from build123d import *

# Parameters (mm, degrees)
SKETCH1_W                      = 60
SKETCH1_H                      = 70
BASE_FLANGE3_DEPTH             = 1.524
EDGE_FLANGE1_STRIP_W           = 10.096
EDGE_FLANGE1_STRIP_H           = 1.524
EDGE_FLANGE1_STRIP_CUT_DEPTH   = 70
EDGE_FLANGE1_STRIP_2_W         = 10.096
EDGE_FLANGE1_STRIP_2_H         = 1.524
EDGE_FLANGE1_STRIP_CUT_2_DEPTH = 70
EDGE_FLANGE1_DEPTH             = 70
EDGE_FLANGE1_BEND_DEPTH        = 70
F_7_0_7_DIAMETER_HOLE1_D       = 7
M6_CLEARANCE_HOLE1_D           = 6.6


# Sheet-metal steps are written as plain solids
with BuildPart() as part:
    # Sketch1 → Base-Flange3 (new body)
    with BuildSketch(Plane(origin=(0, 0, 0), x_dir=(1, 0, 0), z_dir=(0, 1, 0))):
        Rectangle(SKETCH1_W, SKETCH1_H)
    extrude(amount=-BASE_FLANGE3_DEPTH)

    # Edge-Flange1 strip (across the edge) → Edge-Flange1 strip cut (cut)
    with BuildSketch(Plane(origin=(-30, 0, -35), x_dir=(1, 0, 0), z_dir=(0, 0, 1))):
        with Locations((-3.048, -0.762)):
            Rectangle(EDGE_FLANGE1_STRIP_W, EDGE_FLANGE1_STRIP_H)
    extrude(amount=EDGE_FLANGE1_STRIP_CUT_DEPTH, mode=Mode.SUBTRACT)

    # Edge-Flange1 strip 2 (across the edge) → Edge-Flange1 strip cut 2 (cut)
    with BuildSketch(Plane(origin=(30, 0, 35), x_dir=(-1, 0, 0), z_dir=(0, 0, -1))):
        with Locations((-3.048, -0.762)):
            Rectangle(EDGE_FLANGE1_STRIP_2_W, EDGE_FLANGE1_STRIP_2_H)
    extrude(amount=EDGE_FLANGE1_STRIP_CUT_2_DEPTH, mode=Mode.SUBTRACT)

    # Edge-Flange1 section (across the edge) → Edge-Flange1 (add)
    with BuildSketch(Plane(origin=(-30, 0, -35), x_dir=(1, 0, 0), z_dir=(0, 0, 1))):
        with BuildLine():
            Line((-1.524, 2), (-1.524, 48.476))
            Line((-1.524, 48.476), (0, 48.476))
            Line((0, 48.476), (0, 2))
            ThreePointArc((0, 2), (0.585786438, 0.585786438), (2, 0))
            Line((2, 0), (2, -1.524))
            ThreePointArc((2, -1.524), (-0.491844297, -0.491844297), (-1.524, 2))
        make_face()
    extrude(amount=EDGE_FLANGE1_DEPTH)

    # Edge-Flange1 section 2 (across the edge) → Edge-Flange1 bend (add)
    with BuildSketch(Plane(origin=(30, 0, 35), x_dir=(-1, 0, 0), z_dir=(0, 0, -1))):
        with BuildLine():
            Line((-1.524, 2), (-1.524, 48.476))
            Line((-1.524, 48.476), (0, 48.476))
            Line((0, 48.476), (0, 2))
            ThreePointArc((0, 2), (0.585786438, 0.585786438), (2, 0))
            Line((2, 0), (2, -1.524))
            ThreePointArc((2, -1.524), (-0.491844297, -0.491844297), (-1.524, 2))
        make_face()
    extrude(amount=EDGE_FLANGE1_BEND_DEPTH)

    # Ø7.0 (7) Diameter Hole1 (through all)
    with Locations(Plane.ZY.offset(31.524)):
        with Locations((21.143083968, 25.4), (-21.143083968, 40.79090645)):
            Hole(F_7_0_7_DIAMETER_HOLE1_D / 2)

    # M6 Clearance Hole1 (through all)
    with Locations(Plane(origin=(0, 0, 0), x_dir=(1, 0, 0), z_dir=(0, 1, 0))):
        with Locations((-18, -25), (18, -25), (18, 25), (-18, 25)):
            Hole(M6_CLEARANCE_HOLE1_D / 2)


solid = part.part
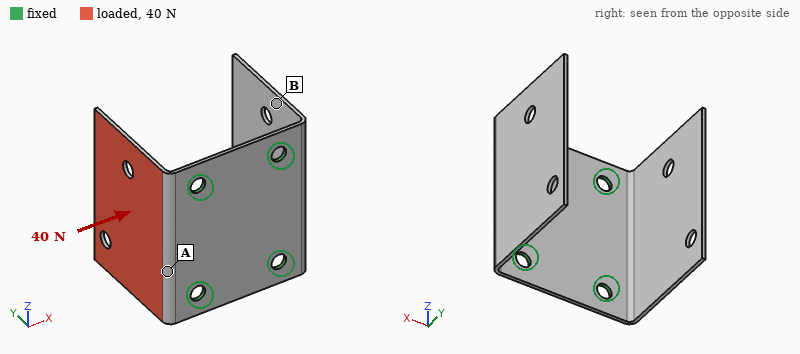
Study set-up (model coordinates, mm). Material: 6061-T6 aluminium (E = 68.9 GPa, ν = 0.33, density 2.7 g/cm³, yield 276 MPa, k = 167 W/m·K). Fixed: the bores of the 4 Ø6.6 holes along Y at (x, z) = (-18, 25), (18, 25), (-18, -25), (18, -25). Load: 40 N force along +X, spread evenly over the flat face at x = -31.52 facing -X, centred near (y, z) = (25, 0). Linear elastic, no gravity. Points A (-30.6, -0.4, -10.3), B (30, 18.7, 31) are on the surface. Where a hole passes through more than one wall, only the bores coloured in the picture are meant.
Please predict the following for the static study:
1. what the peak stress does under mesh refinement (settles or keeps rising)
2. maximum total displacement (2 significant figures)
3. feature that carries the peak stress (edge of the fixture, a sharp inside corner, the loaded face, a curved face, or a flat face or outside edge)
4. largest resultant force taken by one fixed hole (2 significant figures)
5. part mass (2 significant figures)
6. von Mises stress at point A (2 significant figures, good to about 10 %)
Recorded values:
keeps rising
0.77 mm
edge of the fixture
15 N
44 g
29 MPa
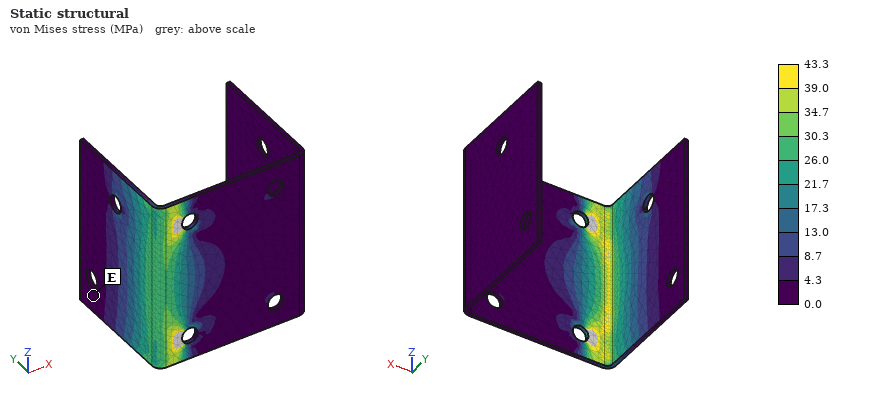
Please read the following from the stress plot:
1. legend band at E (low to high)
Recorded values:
0.0 to 4.3 MPa
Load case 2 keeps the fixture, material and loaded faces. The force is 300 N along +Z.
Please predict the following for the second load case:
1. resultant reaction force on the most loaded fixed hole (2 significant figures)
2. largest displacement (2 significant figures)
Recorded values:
220 N
0.29 mm
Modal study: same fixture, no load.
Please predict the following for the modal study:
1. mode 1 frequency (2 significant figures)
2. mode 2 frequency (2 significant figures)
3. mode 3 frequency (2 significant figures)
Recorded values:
390 Hz
400 Hz
850 Hz
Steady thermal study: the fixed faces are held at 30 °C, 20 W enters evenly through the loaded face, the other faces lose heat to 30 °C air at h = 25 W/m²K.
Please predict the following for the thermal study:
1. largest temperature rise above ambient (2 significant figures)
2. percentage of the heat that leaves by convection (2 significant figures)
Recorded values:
39 K
18 %
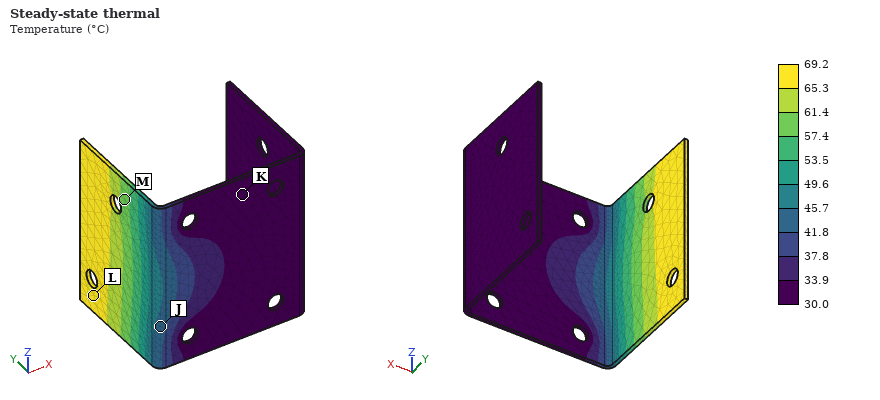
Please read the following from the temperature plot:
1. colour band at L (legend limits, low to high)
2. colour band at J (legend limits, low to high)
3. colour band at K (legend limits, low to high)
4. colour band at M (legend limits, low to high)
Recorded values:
65.3 to 69.2 °C
41.8 to 45.7 °C
30.0 to 33.9 °C
57.4 to 61.4 °C
